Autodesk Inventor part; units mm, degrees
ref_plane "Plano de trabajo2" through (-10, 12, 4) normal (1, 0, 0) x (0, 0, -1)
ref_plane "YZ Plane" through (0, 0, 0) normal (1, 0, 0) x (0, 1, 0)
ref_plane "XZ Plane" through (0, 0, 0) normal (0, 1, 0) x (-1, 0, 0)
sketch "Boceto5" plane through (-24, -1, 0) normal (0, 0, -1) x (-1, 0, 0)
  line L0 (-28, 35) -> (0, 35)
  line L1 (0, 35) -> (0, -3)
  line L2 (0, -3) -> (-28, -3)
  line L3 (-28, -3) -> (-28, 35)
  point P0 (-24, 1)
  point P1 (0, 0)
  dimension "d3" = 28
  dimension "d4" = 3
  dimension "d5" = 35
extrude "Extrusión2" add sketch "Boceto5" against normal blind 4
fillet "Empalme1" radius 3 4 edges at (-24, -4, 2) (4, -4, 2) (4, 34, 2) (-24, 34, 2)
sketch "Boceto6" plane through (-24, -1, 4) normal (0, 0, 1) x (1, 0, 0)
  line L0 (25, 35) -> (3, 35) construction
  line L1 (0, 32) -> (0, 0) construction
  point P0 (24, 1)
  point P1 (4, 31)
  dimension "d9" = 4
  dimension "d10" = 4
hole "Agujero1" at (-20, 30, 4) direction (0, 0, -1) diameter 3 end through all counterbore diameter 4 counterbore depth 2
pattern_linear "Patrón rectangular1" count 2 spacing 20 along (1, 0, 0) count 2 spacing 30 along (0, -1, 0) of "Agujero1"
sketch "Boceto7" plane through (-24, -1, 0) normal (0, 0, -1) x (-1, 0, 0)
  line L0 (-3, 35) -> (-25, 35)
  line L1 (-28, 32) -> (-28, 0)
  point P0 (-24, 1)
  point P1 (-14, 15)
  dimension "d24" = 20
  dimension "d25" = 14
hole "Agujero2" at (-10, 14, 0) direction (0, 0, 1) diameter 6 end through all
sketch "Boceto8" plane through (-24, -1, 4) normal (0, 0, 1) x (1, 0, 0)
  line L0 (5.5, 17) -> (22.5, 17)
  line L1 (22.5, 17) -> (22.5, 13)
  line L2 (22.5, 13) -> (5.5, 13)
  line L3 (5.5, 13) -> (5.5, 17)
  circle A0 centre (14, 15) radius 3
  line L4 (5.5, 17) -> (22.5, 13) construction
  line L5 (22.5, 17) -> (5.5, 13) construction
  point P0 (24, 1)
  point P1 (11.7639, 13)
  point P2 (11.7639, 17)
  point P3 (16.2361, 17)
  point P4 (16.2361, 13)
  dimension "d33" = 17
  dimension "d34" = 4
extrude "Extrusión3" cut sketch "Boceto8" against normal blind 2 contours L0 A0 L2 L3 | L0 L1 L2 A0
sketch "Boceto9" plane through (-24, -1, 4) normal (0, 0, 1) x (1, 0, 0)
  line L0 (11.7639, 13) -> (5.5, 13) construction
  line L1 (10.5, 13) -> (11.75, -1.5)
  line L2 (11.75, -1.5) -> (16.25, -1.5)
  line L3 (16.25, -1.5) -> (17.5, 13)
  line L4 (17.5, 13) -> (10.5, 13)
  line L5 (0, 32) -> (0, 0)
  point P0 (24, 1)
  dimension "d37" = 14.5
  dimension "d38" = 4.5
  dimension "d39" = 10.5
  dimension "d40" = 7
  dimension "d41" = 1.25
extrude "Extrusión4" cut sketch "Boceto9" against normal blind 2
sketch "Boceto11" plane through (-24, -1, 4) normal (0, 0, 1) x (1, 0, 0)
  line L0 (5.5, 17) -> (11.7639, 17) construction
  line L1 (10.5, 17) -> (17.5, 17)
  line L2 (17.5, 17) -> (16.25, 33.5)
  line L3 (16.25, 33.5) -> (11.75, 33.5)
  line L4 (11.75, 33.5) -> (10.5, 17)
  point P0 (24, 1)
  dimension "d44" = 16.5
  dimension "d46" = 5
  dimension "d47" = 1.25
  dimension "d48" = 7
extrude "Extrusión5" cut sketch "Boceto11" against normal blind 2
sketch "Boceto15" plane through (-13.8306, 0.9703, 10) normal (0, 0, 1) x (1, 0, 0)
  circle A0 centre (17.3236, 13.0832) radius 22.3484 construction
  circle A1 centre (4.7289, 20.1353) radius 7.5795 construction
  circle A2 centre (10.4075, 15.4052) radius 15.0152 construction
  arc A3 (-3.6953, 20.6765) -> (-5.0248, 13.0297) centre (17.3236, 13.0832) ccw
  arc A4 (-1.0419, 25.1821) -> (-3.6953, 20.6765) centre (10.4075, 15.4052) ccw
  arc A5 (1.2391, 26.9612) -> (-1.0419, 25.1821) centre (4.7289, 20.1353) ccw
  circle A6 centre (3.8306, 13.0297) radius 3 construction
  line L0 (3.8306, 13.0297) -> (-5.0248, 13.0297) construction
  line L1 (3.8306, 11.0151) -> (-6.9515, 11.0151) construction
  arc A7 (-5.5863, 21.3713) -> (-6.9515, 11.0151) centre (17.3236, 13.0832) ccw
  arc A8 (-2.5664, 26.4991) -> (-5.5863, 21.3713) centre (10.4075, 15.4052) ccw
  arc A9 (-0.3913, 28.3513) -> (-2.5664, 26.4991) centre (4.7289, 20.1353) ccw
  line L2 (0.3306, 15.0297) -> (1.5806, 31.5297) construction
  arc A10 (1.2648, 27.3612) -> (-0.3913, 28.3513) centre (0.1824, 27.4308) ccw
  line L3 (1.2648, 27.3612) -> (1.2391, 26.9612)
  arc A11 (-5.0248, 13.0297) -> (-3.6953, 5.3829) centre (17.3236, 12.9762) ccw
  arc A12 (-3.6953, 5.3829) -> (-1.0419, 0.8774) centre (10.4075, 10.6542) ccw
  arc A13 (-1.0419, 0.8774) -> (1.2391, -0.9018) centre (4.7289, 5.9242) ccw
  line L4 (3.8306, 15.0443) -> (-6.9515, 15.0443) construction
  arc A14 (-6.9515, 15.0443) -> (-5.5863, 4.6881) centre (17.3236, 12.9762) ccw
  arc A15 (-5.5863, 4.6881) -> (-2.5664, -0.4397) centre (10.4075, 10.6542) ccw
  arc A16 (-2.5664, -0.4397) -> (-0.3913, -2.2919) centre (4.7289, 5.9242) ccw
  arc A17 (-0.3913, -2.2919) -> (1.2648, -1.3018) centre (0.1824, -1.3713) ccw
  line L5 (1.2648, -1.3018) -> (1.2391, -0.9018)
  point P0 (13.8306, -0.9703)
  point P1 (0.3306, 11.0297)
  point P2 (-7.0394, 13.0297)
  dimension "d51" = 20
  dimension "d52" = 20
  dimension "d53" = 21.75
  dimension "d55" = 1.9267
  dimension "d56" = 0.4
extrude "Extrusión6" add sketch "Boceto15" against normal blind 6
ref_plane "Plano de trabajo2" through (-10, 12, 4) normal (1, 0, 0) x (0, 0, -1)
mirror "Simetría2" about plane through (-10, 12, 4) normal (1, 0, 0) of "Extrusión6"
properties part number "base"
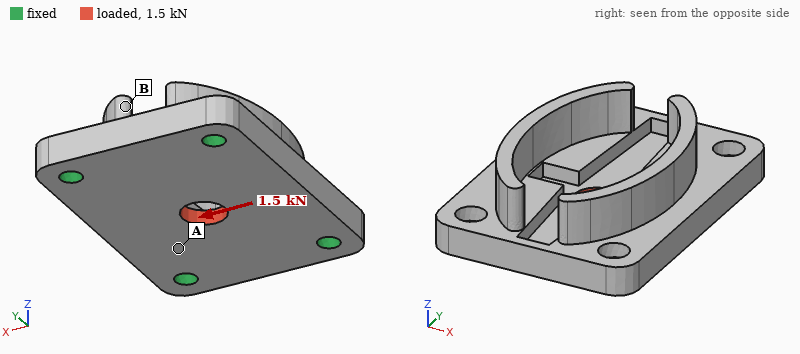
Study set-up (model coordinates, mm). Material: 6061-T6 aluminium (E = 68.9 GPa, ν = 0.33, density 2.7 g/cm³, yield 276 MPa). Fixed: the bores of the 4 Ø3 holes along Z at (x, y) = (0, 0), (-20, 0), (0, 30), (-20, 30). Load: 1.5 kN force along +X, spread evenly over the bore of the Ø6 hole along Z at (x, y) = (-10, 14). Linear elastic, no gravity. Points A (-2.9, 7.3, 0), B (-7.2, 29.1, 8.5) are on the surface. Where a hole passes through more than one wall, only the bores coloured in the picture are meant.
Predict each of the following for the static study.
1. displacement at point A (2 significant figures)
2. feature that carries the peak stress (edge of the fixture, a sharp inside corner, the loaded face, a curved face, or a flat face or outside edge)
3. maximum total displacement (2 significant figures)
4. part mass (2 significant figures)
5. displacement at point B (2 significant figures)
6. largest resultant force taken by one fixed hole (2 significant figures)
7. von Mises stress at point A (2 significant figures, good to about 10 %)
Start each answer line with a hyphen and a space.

- 4.0 µm
- edge of the fixture
- 9.0 µm
- 12 g
- 1.7 µm
- 440 N
- 24 MPa
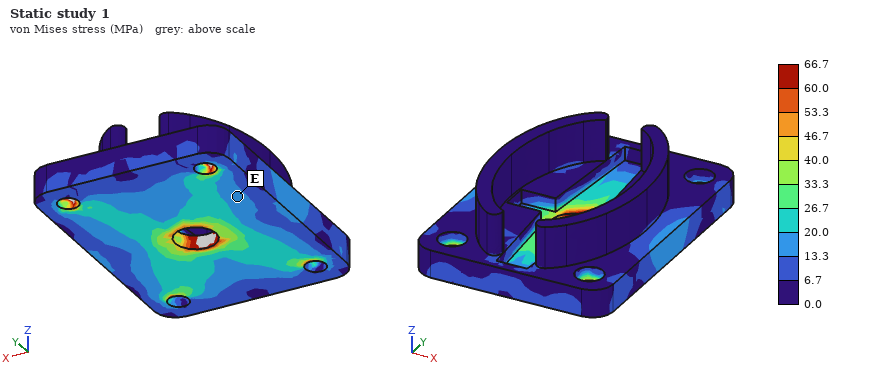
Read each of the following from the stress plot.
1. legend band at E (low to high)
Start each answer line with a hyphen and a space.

- 13.3 to 20.0 MPa
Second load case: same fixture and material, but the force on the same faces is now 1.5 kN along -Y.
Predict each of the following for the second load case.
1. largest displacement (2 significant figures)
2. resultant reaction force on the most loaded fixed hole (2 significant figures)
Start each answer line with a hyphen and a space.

- 5.7 µm
- 410 N
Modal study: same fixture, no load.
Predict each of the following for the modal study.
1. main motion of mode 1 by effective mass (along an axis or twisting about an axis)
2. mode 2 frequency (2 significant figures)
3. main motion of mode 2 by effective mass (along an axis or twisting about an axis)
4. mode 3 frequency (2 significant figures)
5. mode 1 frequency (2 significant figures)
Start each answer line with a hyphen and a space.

- along Z
- 20 kHz
- along Z
- 21 kHz
- 18 kHz
